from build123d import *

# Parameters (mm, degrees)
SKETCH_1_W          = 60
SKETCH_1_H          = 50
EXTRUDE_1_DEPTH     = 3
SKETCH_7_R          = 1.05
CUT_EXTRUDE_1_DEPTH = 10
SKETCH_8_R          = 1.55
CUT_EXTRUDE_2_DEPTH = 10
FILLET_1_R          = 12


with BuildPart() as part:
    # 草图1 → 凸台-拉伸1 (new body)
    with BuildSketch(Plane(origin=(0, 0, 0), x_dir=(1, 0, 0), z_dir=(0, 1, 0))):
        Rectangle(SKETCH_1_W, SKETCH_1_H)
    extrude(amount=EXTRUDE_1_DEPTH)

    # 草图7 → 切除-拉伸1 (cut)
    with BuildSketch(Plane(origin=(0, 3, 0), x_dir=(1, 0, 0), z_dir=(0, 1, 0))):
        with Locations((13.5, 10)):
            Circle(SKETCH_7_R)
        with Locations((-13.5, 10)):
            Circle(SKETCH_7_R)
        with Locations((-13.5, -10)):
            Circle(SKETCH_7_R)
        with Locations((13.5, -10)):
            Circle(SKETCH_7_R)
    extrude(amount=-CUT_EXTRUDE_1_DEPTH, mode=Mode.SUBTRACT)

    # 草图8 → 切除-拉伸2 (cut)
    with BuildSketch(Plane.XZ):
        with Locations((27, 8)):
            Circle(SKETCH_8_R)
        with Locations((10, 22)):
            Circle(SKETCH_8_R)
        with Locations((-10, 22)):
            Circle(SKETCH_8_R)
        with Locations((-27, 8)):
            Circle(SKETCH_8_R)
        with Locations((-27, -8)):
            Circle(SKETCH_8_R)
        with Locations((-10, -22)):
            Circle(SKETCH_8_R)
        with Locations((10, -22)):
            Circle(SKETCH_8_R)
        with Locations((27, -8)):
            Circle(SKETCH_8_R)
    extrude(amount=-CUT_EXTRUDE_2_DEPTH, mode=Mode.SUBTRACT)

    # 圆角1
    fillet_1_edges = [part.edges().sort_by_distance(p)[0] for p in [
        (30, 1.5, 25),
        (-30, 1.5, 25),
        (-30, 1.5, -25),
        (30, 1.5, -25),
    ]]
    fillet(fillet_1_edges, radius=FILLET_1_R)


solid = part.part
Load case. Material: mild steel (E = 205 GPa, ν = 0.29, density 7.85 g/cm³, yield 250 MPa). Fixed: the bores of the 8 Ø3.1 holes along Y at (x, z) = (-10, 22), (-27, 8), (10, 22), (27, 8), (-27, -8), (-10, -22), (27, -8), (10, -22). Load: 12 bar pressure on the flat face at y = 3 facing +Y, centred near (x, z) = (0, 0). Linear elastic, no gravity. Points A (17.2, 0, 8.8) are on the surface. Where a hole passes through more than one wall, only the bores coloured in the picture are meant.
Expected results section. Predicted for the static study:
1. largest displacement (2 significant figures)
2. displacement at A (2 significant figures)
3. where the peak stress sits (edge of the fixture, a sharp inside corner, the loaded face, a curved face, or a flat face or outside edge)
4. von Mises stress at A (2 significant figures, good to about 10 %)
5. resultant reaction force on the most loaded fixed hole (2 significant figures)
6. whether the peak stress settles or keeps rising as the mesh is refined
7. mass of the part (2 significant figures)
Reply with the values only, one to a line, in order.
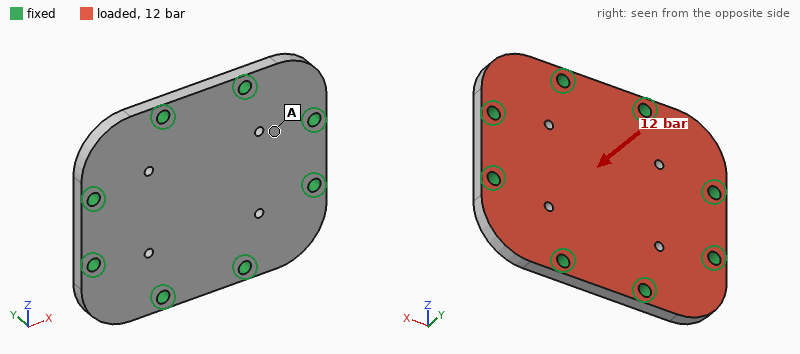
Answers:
19 µm
6.5 µm
edge of the fixture
26 MPa
470 N
keeps rising
66 g
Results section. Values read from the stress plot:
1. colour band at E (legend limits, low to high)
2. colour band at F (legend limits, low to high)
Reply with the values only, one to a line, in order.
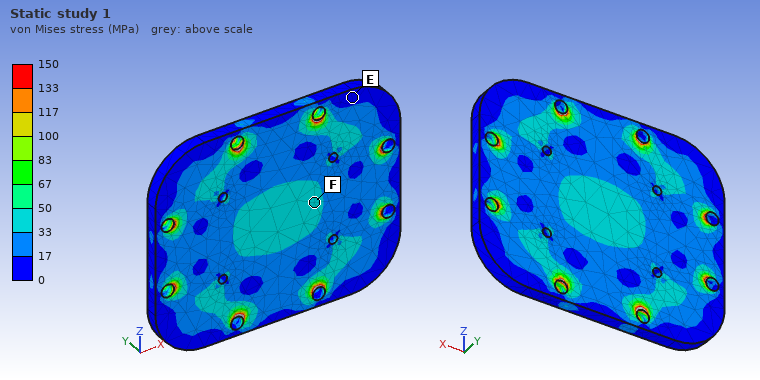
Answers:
0 to 17 MPa
33 to 50 MPa
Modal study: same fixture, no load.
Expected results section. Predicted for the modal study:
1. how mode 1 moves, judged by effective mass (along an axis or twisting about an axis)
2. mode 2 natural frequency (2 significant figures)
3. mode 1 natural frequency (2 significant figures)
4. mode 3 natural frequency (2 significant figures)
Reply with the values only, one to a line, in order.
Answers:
along Y
18 kHz
10 kHz
21 kHz
